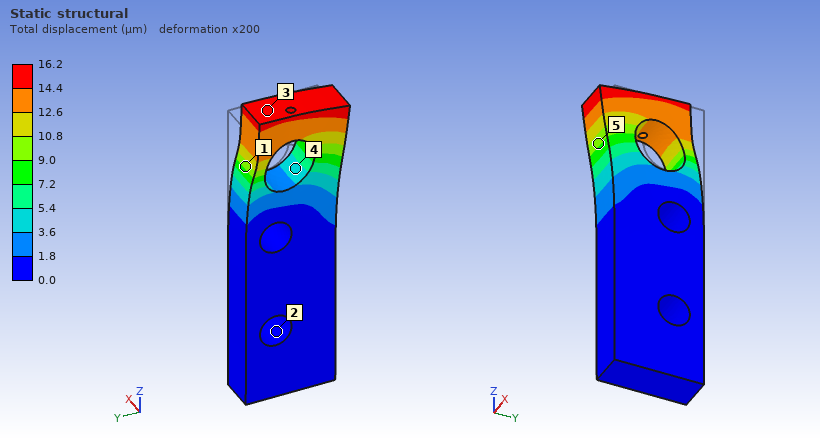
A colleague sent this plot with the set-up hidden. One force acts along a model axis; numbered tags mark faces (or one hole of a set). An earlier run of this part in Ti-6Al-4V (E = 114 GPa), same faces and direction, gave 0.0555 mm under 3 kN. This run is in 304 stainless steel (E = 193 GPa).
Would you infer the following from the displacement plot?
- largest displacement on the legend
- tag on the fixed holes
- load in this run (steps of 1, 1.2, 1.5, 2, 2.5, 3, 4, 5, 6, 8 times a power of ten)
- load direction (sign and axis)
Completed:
16.2 µm
2
1.5 kN
-Y
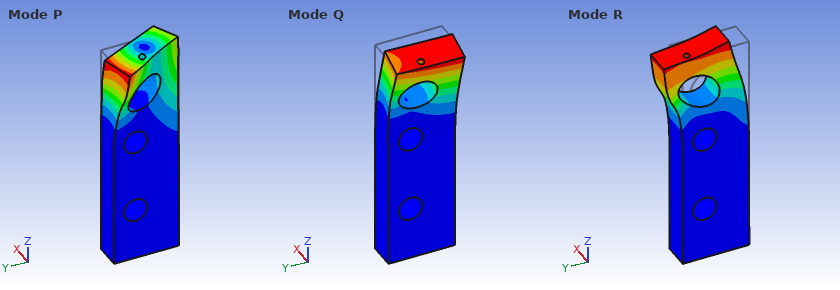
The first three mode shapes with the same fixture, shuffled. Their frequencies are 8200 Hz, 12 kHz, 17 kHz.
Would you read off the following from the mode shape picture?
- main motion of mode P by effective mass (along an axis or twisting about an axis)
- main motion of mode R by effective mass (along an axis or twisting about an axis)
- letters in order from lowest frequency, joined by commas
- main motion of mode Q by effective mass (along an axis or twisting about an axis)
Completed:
twisting about Z
along Y
Q, R, P
along X
